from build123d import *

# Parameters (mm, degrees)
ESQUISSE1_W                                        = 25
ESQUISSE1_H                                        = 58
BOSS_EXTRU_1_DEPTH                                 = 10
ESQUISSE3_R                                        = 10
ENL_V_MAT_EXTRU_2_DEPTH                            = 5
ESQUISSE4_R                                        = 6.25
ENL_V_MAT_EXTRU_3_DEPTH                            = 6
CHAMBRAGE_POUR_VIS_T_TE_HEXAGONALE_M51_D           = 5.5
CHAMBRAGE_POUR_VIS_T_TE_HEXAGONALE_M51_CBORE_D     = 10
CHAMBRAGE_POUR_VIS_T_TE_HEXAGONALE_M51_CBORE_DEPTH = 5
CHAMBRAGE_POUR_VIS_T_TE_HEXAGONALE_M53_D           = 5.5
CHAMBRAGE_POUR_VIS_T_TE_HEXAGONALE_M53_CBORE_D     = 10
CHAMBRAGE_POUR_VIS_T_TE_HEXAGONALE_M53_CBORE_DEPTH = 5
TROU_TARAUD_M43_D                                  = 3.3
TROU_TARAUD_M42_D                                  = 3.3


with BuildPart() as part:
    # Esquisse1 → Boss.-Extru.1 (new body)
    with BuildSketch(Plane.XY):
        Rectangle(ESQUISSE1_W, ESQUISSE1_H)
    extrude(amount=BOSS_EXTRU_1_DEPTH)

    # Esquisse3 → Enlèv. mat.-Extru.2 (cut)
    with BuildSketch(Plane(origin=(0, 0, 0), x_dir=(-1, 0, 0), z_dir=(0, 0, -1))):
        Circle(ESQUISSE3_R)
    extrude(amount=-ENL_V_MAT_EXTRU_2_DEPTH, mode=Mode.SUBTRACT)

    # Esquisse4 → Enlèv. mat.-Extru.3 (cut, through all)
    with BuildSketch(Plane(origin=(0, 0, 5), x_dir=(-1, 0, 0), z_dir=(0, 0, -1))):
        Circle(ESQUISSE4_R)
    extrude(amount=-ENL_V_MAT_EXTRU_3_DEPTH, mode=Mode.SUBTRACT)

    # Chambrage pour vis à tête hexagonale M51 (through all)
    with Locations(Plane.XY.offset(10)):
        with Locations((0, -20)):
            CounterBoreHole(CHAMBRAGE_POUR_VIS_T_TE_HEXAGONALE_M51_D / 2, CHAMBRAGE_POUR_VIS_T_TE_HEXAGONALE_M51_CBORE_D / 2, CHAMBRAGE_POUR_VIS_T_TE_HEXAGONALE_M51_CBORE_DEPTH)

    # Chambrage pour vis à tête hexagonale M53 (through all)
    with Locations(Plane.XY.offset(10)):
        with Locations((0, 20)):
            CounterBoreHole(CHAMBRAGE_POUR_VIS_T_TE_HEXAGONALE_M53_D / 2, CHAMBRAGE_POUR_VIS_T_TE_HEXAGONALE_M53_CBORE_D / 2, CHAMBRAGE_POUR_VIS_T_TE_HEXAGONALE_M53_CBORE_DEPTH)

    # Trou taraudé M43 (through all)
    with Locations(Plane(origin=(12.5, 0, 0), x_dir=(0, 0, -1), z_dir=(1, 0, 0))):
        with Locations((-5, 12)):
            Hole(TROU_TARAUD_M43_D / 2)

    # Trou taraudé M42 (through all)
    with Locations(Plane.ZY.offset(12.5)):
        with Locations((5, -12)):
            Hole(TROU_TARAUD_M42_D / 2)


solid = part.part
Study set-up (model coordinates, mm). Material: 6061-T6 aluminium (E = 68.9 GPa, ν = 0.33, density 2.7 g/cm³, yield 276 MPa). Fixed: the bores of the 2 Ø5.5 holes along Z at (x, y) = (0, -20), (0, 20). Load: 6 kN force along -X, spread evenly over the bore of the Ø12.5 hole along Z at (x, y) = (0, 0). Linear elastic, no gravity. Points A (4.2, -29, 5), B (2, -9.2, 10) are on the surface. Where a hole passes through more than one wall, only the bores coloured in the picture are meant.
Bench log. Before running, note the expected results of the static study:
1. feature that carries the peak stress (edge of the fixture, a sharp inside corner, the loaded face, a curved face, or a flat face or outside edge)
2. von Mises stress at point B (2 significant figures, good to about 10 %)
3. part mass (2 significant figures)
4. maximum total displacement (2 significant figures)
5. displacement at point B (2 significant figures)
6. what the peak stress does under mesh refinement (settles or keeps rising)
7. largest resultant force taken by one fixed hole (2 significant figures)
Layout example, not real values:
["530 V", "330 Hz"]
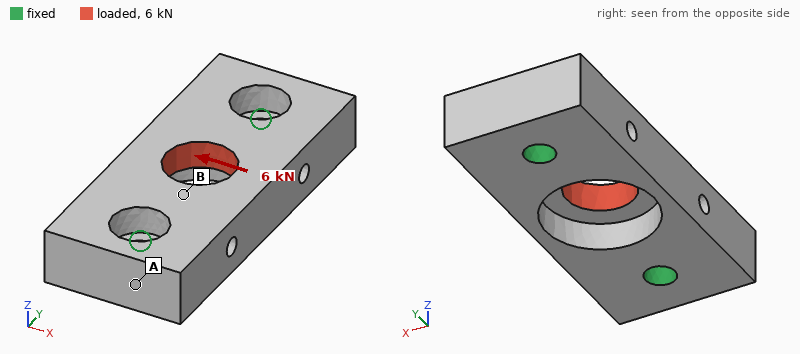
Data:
["edge of the fixture", "62 MPa", "29 g", "53 µm", "32 µm", "keeps rising", "3.0 kN"]
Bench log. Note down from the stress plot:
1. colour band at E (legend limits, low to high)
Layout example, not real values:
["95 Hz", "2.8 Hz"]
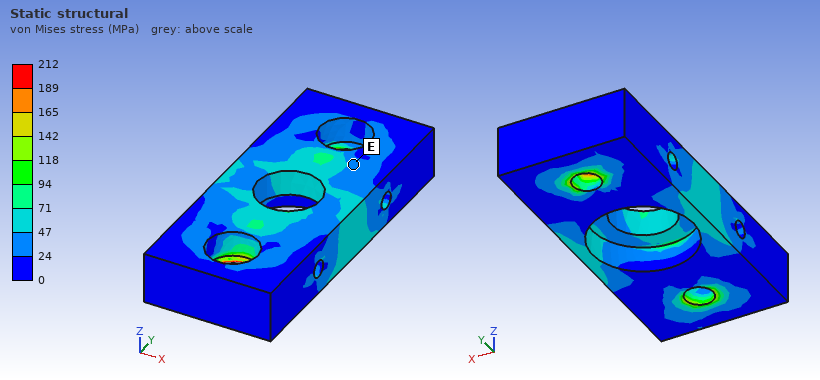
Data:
["24 to 47 MPa"]
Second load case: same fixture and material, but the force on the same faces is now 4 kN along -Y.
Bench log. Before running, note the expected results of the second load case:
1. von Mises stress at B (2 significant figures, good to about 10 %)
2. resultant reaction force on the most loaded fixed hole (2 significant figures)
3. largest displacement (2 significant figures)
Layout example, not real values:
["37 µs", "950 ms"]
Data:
["23 MPa", "2.0 kN", "8.4 µm"]
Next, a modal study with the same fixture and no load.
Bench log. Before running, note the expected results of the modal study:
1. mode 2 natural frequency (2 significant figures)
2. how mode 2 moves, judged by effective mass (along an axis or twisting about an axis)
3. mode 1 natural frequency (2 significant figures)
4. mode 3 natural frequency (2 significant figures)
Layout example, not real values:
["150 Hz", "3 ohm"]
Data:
["18 kHz", "along Z", "13 kHz", "20 kHz"]
